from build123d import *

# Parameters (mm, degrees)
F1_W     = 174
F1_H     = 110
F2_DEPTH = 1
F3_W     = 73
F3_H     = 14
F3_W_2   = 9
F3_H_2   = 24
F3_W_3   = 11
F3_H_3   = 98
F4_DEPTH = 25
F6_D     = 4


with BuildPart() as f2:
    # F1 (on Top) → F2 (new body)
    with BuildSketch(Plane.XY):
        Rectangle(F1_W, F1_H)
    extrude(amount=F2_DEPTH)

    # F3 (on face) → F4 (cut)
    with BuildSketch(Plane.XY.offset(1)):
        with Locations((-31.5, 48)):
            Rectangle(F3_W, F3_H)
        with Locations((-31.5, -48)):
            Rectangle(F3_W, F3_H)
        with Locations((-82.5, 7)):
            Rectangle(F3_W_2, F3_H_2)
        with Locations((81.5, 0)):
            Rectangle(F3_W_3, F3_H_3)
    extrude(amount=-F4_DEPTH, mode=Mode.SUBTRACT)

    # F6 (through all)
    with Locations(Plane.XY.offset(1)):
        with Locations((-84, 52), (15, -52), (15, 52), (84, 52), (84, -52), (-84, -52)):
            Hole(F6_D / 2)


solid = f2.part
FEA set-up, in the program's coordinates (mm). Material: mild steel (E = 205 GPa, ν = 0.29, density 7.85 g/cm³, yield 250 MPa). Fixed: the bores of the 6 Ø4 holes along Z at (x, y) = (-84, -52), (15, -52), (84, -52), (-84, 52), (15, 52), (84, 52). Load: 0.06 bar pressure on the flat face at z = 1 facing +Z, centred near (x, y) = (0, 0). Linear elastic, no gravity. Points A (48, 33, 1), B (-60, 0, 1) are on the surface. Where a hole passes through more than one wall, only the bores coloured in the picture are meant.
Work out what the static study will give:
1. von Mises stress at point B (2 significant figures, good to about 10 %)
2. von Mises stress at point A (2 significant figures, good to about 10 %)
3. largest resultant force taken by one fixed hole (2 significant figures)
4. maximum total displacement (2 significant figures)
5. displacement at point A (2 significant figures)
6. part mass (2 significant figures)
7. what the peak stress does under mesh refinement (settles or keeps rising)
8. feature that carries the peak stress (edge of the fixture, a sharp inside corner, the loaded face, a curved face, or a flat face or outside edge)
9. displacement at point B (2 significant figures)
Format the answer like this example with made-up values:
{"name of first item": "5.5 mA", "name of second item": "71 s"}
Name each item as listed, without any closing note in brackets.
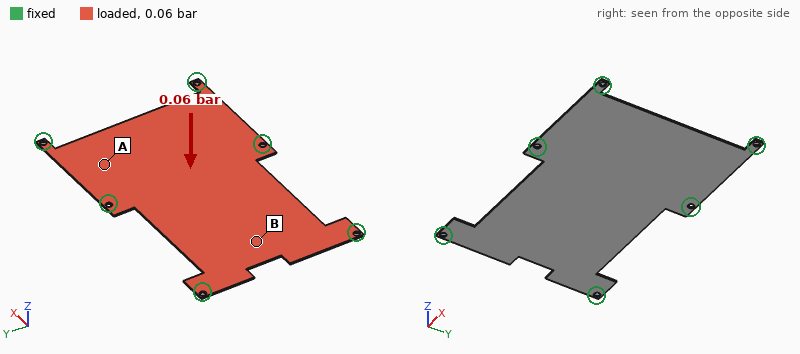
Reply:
{"von Mises stress at point B": "21 MPa", "von Mises stress at point A": "7.3 MPa", "largest resultant force taken by one fixed hole": "26 N", "maximum total displacement": "0.29 mm", "displacement at point A": "0.11 mm", "part mass": "120 g", "what the peak stress does under mesh refinement": "keeps rising", "feature that carries the peak stress": "edge of the fixture", "displacement at point B": "0.26 mm"}
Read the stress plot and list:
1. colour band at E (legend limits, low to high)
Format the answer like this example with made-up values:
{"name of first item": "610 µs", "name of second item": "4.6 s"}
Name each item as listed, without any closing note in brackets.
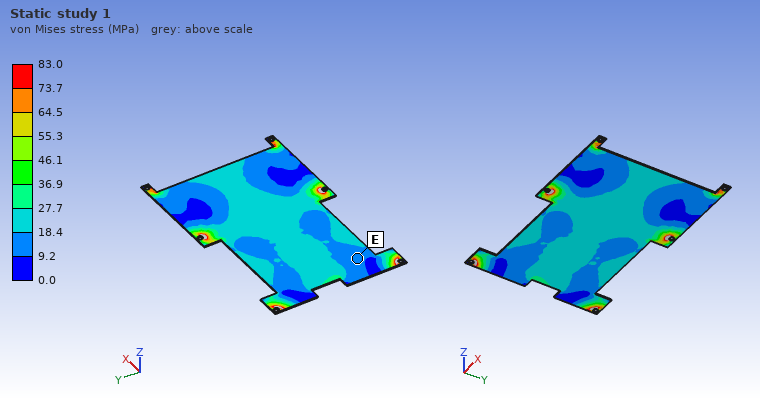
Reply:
{"colour band at E": "9.2 to 18.4 MPa"}
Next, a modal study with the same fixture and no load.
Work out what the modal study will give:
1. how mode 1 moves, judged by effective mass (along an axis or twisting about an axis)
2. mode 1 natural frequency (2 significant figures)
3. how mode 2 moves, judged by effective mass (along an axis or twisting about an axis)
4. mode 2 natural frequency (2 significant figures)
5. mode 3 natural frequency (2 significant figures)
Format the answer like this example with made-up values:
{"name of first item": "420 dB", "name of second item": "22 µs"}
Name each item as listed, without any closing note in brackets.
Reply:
{"how mode 1 moves, judged by effective mass": "along Z", "mode 1 natural frequency": "300 Hz", "how mode 2 moves, judged by effective mass": "along Z", "mode 2 natural frequency": "370 Hz", "mode 3 natural frequency": "600 Hz"}
